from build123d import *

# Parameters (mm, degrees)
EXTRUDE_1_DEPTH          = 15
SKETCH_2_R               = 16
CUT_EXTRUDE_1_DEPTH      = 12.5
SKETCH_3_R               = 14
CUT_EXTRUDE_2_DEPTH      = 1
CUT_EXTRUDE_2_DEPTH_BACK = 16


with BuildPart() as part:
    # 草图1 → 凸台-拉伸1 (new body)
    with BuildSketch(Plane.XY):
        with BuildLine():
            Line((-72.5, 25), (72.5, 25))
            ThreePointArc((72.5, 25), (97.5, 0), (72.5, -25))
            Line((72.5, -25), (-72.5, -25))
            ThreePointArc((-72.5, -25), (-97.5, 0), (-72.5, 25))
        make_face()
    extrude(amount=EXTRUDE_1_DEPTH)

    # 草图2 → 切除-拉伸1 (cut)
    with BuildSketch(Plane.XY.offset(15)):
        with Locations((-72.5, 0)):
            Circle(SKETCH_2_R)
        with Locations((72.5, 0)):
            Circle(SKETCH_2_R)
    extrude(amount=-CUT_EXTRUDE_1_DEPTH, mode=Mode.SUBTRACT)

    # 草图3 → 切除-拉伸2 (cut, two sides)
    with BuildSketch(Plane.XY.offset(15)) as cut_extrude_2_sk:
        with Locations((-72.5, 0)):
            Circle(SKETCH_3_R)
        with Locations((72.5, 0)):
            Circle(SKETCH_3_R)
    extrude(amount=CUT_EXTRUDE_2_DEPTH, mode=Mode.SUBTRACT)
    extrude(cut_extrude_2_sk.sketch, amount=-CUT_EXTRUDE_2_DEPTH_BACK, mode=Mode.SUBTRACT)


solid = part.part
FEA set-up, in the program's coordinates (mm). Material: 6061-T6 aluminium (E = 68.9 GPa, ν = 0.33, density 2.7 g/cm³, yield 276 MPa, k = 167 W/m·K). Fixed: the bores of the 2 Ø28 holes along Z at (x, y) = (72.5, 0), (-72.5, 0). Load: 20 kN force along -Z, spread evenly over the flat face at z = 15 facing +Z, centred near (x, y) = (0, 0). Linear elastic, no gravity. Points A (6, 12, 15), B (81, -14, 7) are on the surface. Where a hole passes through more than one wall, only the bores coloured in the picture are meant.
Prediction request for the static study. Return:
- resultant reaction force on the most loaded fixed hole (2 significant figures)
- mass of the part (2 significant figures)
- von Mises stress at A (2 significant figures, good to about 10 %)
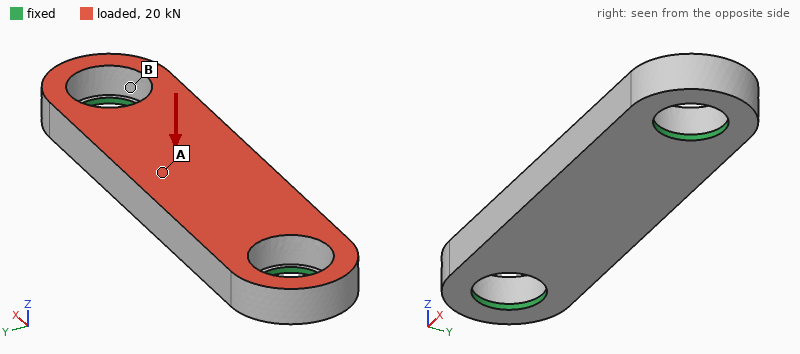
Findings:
14 kN
310 g
73 MPa
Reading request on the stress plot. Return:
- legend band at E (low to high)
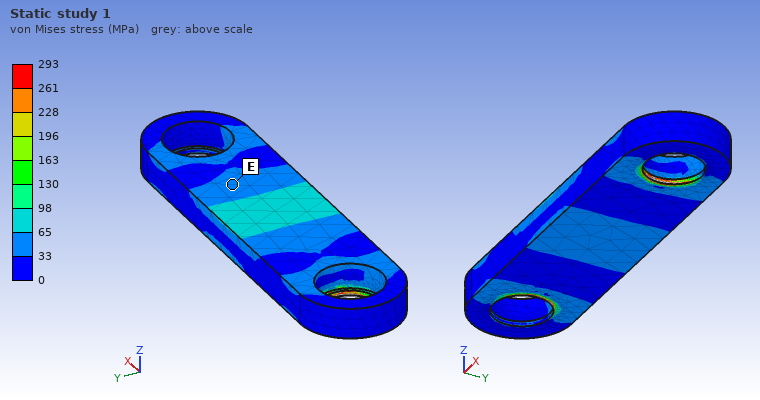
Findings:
33 to 65 MPa
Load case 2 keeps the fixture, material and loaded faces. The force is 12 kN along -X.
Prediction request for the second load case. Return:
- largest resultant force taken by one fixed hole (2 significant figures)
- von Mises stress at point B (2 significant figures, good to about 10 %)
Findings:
6.1 kN
17 MPa
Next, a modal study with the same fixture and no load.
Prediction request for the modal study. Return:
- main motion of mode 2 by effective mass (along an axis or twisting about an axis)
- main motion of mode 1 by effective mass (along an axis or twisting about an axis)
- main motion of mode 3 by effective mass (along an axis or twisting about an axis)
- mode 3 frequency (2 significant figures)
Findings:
along Y
along Z
along Y
6600 Hz
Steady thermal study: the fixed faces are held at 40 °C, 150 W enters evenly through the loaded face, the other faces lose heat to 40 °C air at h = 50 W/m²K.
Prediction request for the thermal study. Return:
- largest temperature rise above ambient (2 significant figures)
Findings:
24 K
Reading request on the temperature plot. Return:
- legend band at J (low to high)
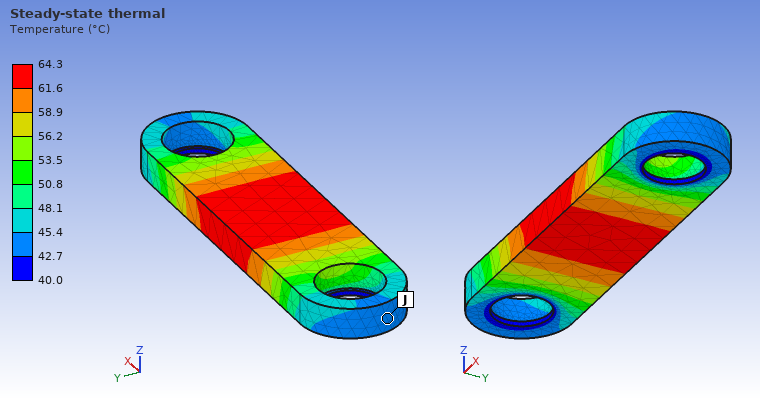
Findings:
42.7 to 45.4 °C
